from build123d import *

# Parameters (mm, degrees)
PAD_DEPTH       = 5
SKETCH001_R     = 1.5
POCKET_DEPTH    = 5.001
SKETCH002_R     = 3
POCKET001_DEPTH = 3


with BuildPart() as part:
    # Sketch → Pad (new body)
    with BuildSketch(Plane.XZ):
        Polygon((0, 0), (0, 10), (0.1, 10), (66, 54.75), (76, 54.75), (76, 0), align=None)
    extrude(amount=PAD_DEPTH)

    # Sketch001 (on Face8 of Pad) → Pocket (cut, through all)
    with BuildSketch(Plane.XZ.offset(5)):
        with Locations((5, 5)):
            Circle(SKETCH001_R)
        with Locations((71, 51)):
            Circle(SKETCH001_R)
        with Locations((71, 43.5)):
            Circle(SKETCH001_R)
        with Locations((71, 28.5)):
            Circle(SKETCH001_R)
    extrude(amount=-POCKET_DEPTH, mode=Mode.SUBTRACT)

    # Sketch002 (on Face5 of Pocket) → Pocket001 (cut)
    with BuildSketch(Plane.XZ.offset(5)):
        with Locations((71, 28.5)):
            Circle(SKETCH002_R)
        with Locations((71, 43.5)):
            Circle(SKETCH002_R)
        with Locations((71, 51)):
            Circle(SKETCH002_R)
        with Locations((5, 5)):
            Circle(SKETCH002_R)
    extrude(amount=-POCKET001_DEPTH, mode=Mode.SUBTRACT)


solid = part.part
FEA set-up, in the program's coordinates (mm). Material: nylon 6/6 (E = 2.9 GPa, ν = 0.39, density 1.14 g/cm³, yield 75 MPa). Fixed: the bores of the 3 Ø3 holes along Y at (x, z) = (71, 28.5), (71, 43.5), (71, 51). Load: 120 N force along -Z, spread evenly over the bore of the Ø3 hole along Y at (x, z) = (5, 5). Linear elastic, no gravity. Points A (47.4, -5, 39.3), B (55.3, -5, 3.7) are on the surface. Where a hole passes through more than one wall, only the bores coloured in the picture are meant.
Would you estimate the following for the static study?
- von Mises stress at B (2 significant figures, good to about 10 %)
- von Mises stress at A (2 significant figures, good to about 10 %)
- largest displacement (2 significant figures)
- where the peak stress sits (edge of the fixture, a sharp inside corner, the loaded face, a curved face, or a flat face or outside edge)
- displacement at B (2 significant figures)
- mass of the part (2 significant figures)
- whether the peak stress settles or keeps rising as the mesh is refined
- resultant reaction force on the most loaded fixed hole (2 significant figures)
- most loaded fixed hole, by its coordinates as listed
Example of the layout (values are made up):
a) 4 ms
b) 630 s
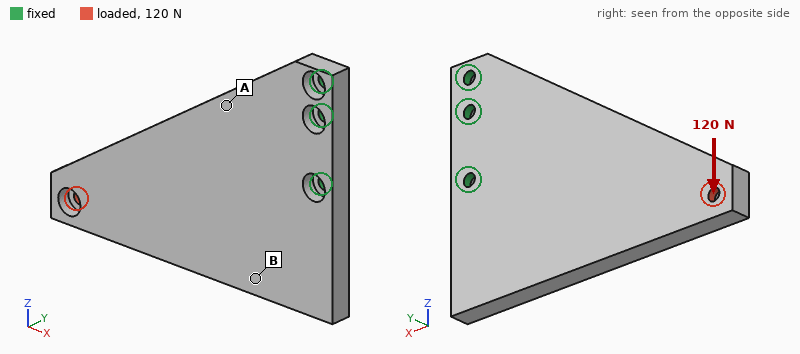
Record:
a) 2.2 MPa
b) 4.6 MPa
c) 0.99 mm
d) edge of the fixture
e) 0.37 mm
f) 15 g
g) keeps rising
h) 370 N
i) (71, 28.5)
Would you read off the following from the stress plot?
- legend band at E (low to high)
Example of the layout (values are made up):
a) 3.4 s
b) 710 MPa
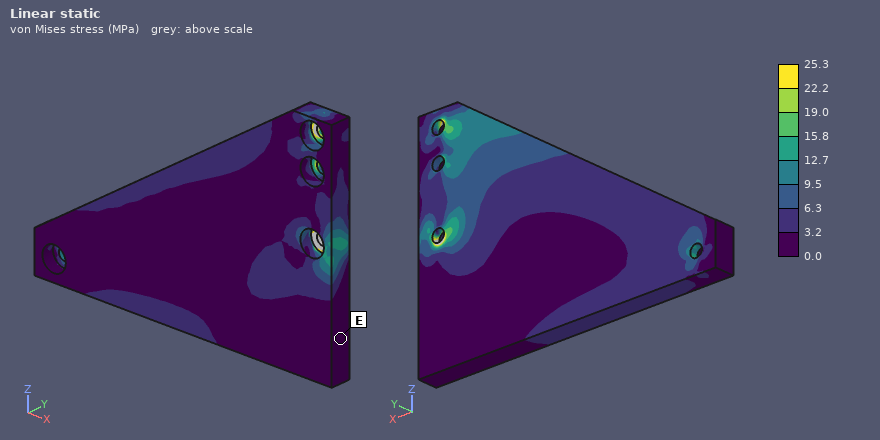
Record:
a) 0.0 to 3.2 MPa
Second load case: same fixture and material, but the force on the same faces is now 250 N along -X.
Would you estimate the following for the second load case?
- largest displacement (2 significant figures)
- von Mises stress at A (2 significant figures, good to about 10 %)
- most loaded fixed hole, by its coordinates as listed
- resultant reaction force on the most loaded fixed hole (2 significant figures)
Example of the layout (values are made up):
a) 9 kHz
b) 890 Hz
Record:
a) 0.93 mm
b) 5.2 MPa
c) (71, 28.5)
d) 510 N
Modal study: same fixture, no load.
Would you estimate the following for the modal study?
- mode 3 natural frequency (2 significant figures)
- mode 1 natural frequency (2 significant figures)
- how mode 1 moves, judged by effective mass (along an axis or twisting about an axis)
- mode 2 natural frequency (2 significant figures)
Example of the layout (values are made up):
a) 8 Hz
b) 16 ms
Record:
a) 1200 Hz
b) 230 Hz
c) along Y
d) 970 Hz
